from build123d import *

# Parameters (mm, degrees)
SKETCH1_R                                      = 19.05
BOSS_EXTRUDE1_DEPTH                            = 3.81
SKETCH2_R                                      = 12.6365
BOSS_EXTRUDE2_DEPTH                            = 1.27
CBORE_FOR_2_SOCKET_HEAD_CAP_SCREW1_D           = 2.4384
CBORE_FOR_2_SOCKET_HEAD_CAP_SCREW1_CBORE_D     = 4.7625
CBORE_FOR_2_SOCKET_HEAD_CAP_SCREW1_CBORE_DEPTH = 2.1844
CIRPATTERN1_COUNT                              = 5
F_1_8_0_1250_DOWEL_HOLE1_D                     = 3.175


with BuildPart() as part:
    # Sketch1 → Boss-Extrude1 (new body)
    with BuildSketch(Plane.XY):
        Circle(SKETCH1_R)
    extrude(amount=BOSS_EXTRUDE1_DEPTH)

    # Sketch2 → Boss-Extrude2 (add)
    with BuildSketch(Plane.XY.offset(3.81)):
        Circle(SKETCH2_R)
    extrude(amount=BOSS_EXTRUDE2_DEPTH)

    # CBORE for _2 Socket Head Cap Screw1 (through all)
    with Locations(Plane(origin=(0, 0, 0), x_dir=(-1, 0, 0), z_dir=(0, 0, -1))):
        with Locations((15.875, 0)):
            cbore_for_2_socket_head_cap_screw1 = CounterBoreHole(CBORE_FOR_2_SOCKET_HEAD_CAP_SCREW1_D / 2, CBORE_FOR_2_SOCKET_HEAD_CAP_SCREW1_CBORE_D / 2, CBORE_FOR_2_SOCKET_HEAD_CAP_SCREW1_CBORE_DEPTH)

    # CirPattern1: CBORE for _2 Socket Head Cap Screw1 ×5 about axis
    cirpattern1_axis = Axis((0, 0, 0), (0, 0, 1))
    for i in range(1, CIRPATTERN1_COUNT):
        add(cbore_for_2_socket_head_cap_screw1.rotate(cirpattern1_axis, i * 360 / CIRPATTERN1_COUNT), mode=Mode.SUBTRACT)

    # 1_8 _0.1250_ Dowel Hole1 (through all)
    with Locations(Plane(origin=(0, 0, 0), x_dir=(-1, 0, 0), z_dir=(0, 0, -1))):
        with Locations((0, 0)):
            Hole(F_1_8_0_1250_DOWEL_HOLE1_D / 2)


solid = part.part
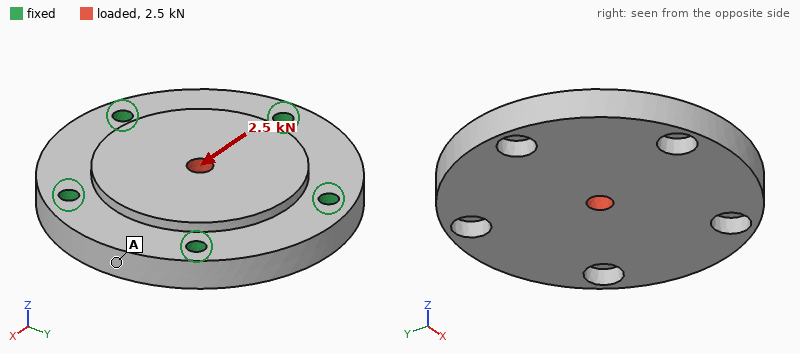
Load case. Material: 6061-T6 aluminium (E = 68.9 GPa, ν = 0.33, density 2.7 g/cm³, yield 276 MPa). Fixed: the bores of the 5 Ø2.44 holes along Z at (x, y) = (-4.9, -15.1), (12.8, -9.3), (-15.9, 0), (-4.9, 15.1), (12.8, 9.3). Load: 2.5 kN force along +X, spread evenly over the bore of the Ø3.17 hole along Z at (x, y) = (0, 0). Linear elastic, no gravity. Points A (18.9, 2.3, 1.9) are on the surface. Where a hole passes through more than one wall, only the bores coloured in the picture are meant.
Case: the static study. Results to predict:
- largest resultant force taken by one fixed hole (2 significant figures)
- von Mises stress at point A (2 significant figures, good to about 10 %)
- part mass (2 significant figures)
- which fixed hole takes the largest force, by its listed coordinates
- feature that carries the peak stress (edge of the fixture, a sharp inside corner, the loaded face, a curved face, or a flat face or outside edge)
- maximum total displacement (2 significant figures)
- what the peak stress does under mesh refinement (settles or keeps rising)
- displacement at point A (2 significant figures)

660 N
12 MPa
13 g
(-15.9, 0)
edge of the fixture
7.0 µm
keeps rising
3.3 µm
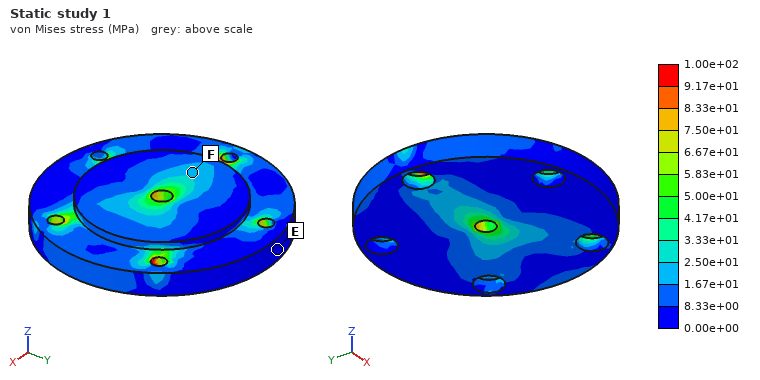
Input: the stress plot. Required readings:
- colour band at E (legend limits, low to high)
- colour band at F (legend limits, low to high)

0.00e+00 to 8.33e+00 MPa
1.67e+01 to 2.50e+01 MPa
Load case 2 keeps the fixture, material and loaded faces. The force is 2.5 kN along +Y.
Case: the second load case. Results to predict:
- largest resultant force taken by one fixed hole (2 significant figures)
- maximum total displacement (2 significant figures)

640 N
7.0 µm
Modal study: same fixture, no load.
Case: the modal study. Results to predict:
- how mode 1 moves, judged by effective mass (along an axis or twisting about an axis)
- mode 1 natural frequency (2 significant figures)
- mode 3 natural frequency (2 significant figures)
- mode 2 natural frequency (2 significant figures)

along Z
23 kHz
32 kHz
32 kHz
